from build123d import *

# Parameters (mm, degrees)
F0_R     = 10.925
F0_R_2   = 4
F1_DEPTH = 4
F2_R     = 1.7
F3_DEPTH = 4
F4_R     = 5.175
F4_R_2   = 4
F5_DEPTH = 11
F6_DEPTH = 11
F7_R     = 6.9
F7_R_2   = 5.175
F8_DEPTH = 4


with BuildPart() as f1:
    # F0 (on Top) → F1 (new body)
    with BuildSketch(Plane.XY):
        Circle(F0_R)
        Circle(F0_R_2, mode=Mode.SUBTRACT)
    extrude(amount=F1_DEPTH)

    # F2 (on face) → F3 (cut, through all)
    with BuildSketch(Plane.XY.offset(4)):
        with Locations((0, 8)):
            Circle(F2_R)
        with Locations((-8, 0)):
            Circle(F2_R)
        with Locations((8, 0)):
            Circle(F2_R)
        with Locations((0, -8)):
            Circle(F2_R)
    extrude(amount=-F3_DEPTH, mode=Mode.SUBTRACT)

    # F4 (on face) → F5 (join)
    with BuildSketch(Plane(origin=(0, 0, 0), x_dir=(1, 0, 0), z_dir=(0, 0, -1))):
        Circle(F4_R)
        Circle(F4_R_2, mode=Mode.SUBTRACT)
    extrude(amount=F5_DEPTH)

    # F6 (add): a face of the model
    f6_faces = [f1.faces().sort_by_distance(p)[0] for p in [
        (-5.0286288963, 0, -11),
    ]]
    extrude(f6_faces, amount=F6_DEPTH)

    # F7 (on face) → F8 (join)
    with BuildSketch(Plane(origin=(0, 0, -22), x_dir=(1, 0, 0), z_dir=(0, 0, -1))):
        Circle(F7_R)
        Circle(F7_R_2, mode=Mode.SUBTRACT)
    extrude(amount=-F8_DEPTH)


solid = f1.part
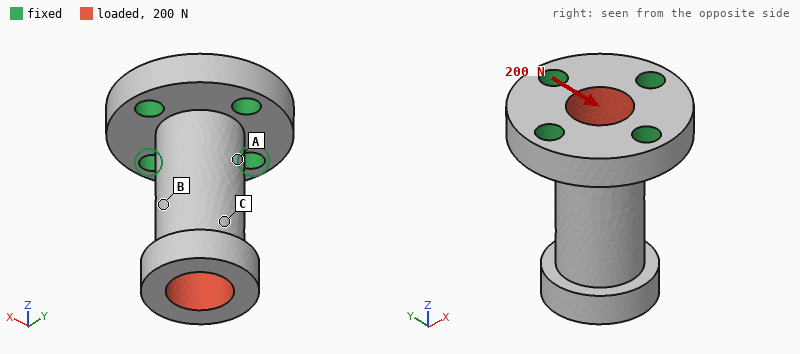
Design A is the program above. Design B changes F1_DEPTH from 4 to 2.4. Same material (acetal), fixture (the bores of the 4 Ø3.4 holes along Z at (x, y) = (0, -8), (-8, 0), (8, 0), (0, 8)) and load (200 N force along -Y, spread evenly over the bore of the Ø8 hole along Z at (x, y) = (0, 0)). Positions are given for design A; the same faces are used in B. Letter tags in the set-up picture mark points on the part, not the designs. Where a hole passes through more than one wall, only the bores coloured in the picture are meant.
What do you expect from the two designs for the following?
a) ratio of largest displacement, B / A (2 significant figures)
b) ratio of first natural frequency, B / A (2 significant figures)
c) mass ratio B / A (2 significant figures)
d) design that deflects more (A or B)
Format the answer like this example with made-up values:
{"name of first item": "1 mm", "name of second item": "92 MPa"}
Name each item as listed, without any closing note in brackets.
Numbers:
{"ratio of largest displacement, B / A": "1.3", "ratio of first natural frequency, B / A": "0.92", "mass ratio B / A": "0.79", "design that deflects more": "B"}
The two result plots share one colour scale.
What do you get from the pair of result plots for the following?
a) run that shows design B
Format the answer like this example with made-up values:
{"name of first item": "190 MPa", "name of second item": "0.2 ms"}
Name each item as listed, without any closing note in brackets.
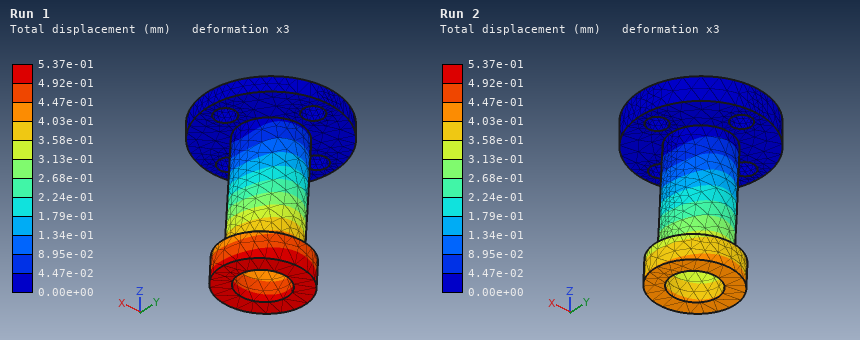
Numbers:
{"run that shows design B": "Run 1"}
